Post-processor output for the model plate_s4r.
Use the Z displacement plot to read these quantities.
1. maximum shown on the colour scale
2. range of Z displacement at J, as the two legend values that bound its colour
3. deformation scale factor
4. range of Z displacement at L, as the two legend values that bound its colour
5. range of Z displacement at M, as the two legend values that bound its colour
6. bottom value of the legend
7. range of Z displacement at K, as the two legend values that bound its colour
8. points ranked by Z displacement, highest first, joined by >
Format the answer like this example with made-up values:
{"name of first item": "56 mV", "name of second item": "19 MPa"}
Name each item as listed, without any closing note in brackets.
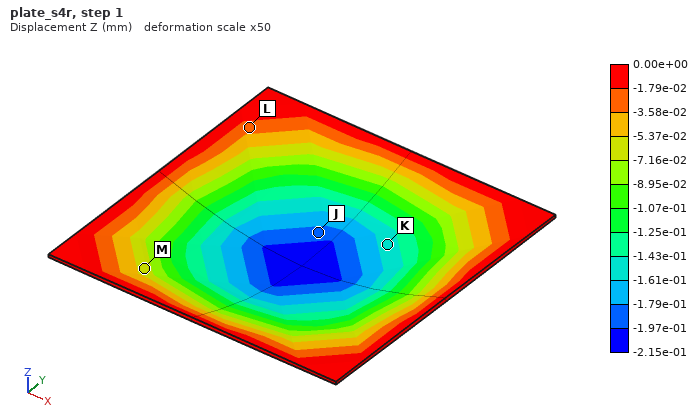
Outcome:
{"maximum shown on the colour scale": "0.00e+00 mm", "range of Z displacement at J, as the two legend values that bound its colour": "-1.97e-01 to -1.79e-01 mm", "deformation scale factor": "50", "range of Z displacement at L, as the two legend values that bound its colour": "-3.58e-02 to -1.79e-02 mm", "range of Z displacement at M, as the two legend values that bound its colour": "-7.16e-02 to -5.37e-02 mm", "bottom value of the legend": "-2.15e-01 mm", "range of Z displacement at K, as the two legend values that bound its colour": "-1.61e-01 to -1.43e-01 mm", "points ranked by Z displacement, highest first, joined by >": "L > M > K > J"}
